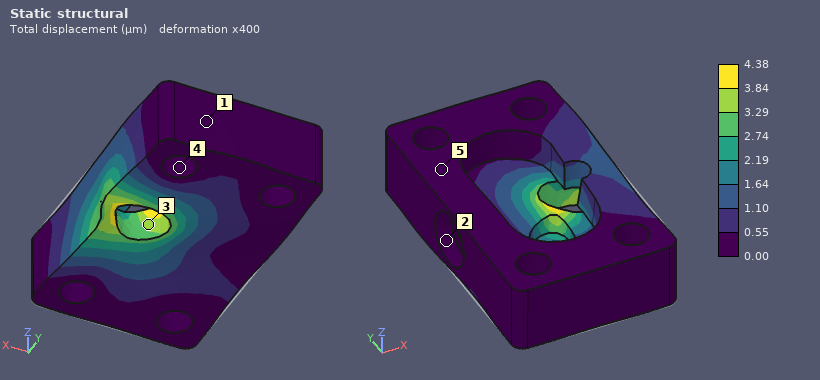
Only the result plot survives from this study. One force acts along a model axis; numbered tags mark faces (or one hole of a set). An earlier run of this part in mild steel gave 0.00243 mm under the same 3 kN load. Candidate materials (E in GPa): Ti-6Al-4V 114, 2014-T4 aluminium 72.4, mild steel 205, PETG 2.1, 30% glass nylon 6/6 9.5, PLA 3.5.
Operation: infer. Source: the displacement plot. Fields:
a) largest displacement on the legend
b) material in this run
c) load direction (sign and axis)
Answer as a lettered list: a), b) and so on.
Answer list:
a) 4.38 µm
b) Ti-6Al-4V
c) +Y
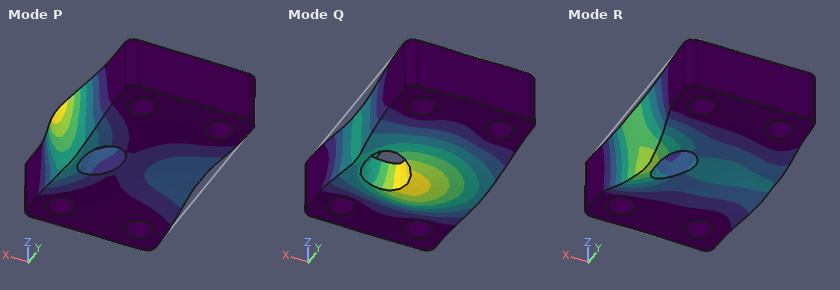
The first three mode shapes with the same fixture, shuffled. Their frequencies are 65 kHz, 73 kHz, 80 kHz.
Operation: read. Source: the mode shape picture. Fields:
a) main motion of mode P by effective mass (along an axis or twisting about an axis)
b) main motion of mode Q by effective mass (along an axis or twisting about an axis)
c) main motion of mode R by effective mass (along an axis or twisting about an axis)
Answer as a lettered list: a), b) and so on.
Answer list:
a) along X
b) along Z
c) along X
